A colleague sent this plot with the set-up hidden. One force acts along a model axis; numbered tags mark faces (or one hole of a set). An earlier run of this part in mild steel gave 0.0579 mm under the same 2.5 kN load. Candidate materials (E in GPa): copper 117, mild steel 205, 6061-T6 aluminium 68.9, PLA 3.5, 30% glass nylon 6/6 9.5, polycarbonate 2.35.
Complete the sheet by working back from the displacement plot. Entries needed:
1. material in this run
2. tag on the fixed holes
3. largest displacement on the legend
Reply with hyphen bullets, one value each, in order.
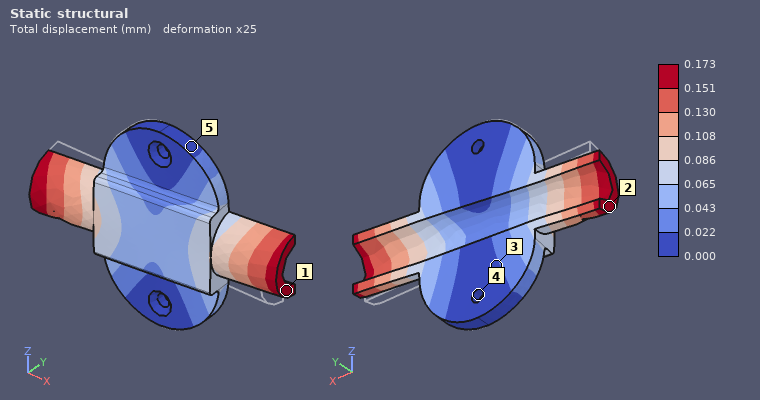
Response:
- 6061-T6 aluminium
- 4
- 0.173 mm
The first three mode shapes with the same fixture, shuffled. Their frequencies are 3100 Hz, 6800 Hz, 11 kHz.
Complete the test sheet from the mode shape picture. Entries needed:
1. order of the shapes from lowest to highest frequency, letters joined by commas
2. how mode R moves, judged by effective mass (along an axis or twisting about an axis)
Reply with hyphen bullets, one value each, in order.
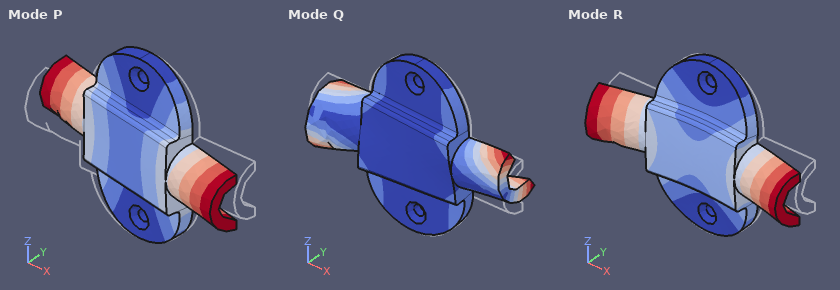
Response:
- P, R, Q
- along Y
